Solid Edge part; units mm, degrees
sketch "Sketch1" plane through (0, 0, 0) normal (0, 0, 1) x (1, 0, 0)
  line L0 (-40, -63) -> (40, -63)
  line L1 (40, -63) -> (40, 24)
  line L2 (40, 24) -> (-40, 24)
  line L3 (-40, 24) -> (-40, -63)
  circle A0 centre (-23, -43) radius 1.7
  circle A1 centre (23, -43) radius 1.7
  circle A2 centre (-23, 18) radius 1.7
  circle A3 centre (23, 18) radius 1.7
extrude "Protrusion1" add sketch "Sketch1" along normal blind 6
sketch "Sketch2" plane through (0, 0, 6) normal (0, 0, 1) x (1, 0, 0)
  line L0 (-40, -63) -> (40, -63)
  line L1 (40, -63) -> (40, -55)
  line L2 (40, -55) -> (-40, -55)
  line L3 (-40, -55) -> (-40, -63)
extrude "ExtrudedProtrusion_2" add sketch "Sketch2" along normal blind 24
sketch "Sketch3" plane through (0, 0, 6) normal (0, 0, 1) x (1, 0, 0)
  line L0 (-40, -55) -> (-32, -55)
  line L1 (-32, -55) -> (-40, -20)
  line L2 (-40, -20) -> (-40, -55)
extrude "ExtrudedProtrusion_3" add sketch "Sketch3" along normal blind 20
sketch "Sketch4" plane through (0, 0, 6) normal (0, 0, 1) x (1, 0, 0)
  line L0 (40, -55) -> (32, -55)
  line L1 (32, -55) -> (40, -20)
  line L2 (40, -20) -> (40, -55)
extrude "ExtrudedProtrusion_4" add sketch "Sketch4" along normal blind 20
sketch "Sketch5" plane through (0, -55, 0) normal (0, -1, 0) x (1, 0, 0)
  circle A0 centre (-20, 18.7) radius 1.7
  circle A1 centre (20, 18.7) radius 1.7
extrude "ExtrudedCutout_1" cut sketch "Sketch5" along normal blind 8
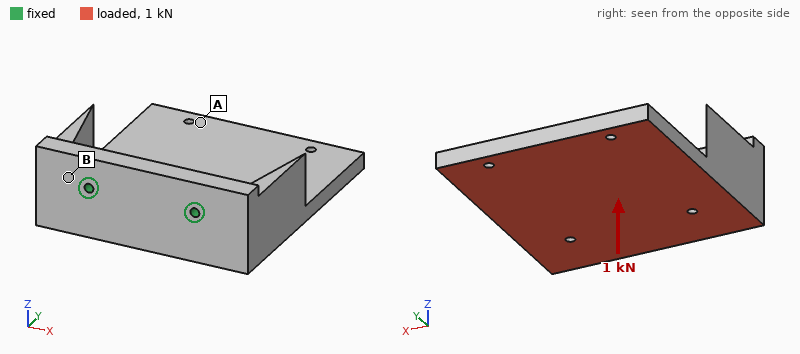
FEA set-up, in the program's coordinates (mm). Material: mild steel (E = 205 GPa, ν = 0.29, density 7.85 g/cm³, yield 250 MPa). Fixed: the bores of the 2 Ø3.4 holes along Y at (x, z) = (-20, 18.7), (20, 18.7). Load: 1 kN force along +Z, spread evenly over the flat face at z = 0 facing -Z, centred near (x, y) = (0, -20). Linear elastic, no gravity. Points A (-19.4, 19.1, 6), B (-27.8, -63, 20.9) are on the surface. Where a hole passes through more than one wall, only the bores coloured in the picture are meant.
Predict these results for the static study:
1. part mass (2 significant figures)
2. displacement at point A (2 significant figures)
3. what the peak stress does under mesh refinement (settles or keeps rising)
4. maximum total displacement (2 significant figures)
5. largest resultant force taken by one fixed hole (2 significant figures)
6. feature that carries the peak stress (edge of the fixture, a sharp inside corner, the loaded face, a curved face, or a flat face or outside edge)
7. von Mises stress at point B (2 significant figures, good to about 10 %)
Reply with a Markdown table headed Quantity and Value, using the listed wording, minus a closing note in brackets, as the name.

| Quantity | Value |
|---|---|
| part mass | 490 g |
| displacement at point A | 0.15 mm |
| what the peak stress does under mesh refinement | keeps rising |
| maximum total displacement | 0.17 mm |
| largest resultant force taken by one fixed hole | 500 N |
| feature that carries the peak stress | edge of the fixture |
| von Mises stress at point B | 32 MPa |
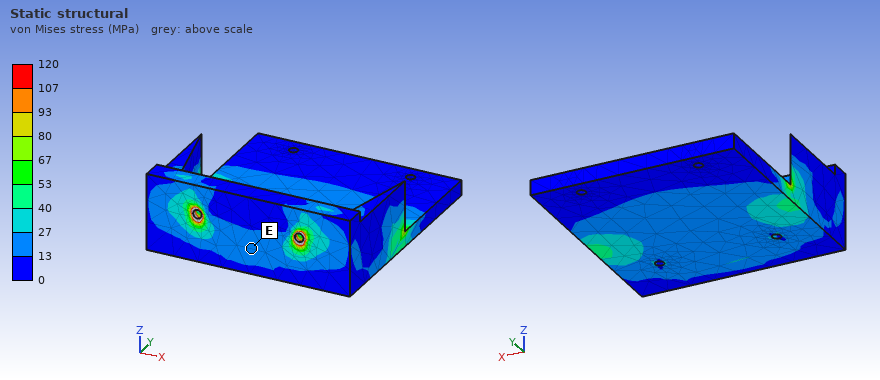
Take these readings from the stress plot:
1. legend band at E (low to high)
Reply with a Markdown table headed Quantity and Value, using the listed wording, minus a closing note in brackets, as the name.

| Quantity | Value |
|---|---|
| legend band at E | 13 to 27 MPa |
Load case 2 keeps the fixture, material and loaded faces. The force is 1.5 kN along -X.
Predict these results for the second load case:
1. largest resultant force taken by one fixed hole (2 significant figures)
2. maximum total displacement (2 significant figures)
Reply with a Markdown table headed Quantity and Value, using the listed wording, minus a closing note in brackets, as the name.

| Quantity | Value |
|---|---|
| largest resultant force taken by one fixed hole | 1.6 kN |
| maximum total displacement | 32 µm |
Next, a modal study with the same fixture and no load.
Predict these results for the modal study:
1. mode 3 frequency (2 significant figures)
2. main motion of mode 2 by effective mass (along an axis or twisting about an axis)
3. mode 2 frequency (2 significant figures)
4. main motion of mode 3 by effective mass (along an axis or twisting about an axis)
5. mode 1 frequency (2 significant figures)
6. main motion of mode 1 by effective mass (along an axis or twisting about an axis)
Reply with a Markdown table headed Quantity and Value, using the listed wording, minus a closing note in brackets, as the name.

| Quantity | Value |
|---|---|
| mode 3 frequency | 2900 Hz |
| main motion of mode 2 by effective mass | along X |
| mode 2 frequency | 1800 Hz |
| main motion of mode 3 by effective mass | along X |
| mode 1 frequency | 850 Hz |
| main motion of mode 1 by effective mass | along Z |
